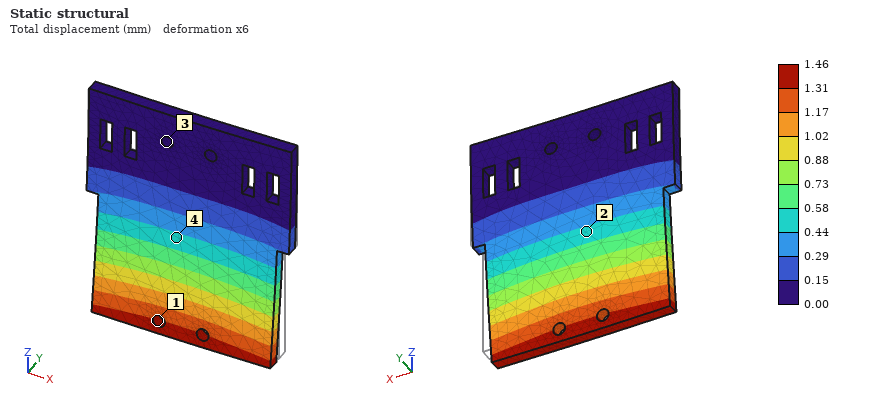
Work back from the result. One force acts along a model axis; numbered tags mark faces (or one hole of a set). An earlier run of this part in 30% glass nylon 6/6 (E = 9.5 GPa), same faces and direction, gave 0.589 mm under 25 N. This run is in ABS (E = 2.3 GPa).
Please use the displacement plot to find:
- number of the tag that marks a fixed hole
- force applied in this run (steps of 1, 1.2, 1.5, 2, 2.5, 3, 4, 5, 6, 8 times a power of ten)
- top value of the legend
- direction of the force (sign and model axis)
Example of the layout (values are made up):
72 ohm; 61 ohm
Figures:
3; 15 N; 1.46 mm; -Y
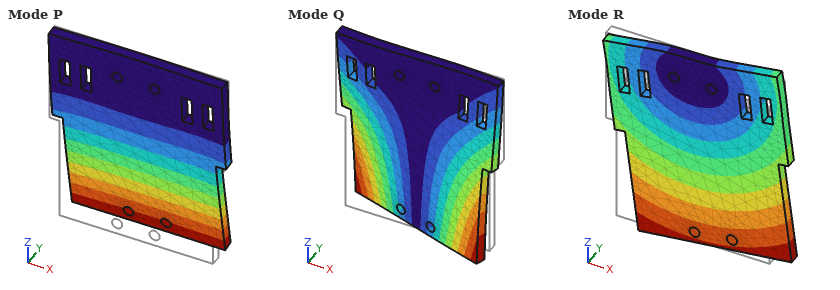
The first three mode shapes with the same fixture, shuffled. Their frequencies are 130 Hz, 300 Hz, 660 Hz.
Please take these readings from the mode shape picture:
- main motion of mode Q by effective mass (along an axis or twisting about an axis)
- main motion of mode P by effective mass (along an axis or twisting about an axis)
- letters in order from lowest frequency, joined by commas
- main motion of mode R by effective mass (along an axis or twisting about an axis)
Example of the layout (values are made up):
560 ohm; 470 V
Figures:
twisting about Z; along Y; P, Q, R; along X
